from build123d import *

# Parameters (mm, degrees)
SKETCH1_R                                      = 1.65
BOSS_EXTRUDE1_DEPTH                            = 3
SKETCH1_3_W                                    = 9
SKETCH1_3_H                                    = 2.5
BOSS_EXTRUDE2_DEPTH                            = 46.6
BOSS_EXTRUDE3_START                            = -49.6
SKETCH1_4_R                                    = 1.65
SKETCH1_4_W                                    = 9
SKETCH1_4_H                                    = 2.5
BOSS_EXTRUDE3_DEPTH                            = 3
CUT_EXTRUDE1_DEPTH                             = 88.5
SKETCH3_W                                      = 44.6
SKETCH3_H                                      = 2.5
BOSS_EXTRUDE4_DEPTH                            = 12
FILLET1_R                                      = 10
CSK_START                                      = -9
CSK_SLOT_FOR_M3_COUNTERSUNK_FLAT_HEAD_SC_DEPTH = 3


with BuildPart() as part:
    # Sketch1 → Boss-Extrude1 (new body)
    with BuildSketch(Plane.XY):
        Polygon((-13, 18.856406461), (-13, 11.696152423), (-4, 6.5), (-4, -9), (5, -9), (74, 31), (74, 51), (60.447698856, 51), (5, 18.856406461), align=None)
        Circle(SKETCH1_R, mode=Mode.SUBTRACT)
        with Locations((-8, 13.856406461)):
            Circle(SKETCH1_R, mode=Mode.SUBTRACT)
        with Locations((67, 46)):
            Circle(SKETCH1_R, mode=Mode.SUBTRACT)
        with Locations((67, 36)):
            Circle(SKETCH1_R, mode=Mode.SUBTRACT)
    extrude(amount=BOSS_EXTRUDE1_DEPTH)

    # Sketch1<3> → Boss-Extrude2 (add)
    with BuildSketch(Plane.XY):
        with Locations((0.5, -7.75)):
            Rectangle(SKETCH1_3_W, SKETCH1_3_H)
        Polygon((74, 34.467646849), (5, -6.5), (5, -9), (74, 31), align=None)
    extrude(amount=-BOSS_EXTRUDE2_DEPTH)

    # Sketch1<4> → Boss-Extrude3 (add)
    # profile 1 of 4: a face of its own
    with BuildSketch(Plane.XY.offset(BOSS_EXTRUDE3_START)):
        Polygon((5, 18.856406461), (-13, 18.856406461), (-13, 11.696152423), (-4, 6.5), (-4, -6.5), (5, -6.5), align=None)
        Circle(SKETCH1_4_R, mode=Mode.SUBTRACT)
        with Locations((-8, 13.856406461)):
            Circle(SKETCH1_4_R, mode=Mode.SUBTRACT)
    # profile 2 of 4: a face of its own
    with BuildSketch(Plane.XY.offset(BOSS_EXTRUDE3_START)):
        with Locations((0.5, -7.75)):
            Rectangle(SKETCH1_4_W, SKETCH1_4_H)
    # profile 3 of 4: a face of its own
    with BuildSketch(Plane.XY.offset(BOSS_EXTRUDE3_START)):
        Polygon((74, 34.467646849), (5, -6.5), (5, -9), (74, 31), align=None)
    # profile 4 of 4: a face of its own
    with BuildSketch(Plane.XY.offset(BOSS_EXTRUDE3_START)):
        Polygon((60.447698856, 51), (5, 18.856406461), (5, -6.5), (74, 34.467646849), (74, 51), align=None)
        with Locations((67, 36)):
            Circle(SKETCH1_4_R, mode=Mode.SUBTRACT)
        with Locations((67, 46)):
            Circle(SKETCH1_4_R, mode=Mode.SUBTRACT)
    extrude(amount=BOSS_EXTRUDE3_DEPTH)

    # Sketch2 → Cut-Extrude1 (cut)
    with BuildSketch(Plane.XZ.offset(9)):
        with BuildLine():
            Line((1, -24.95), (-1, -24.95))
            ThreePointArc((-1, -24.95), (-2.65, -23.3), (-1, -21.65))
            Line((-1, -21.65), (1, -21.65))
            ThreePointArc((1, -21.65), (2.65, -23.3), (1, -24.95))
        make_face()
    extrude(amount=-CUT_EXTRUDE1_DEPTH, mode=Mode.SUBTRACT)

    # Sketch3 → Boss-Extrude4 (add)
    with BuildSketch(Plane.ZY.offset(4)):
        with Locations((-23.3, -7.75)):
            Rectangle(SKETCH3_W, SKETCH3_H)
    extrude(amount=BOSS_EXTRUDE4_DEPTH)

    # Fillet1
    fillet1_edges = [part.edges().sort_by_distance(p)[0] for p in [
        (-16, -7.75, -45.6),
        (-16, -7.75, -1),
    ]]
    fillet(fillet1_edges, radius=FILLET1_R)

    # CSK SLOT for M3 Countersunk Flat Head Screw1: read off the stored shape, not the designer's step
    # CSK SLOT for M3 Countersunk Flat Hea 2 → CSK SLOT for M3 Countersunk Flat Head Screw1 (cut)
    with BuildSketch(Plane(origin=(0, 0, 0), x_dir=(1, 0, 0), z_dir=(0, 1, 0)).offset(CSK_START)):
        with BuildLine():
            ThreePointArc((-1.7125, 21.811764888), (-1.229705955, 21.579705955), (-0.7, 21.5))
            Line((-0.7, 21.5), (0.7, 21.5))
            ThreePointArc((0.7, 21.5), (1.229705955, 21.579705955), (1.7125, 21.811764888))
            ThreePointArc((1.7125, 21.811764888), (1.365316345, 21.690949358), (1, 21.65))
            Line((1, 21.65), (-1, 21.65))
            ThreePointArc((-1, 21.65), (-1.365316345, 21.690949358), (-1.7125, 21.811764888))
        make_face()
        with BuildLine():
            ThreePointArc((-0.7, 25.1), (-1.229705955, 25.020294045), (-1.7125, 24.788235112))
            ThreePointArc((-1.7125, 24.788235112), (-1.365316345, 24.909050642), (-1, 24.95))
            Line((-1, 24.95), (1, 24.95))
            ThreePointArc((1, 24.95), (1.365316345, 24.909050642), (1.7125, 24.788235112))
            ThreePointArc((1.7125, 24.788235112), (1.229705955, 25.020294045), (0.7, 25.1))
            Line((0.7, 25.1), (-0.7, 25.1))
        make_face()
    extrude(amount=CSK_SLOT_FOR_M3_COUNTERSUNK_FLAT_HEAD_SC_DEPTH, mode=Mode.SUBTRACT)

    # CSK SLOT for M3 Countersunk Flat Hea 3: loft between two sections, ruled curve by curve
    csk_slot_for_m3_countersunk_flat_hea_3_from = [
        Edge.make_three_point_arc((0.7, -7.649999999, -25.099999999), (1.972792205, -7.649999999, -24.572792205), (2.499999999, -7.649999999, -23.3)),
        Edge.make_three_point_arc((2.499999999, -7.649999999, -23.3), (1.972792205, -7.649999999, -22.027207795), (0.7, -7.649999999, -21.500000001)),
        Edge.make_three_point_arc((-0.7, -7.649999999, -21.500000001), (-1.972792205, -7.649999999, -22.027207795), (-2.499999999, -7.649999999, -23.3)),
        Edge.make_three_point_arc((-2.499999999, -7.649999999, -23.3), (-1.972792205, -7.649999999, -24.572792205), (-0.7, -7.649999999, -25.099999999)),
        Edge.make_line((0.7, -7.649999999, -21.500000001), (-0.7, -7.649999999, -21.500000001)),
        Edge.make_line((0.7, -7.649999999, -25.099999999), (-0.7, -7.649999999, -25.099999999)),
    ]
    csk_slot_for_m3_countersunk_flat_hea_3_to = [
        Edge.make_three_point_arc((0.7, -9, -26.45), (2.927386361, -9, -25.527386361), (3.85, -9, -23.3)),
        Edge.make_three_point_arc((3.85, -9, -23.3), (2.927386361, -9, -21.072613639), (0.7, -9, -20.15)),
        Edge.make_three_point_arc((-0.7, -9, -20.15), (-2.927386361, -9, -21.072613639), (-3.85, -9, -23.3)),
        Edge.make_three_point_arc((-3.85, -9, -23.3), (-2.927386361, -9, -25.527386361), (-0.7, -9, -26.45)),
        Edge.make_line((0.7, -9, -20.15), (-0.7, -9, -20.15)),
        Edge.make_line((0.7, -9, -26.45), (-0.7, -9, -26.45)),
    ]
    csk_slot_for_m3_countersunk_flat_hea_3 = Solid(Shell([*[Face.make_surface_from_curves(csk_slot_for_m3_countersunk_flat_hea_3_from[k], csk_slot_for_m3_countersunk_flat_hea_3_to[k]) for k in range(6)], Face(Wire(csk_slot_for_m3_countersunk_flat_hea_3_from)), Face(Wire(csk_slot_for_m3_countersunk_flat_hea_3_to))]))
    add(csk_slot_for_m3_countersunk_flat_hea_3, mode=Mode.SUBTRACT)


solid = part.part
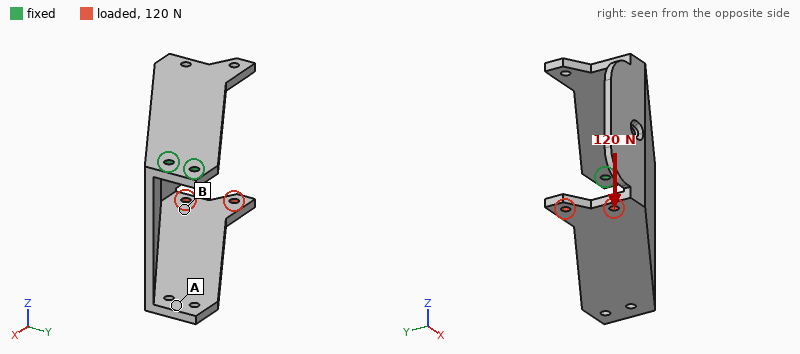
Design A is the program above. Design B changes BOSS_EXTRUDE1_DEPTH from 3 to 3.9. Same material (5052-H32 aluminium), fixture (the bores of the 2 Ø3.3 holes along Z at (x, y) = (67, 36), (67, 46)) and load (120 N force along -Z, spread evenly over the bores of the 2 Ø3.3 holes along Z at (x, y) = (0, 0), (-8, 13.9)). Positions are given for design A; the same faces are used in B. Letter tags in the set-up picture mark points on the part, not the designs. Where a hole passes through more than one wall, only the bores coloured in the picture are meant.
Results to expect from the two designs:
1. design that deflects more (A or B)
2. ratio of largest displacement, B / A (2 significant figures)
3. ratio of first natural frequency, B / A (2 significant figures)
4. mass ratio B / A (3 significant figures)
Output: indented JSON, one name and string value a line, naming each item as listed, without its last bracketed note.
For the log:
{
  "design that deflects more": "A",
  "ratio of largest displacement, B / A": "0.68",
  "ratio of first natural frequency, B / A": "1.2",
  "mass ratio B / A": "1.08"
}
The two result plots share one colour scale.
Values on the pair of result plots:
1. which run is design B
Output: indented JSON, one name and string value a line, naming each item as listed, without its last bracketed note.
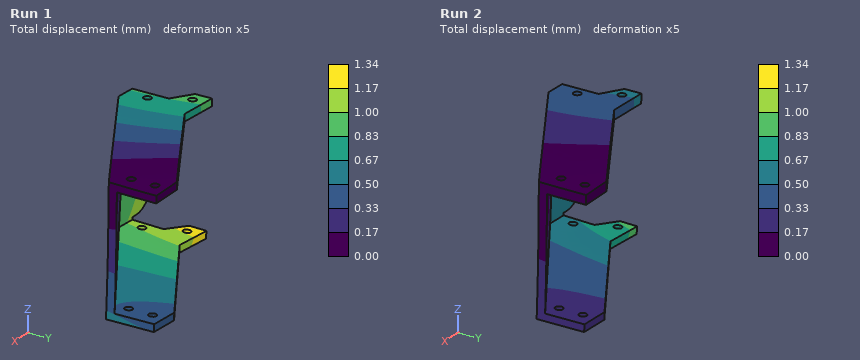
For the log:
{
  "which run is design B": "Run 2"
}
